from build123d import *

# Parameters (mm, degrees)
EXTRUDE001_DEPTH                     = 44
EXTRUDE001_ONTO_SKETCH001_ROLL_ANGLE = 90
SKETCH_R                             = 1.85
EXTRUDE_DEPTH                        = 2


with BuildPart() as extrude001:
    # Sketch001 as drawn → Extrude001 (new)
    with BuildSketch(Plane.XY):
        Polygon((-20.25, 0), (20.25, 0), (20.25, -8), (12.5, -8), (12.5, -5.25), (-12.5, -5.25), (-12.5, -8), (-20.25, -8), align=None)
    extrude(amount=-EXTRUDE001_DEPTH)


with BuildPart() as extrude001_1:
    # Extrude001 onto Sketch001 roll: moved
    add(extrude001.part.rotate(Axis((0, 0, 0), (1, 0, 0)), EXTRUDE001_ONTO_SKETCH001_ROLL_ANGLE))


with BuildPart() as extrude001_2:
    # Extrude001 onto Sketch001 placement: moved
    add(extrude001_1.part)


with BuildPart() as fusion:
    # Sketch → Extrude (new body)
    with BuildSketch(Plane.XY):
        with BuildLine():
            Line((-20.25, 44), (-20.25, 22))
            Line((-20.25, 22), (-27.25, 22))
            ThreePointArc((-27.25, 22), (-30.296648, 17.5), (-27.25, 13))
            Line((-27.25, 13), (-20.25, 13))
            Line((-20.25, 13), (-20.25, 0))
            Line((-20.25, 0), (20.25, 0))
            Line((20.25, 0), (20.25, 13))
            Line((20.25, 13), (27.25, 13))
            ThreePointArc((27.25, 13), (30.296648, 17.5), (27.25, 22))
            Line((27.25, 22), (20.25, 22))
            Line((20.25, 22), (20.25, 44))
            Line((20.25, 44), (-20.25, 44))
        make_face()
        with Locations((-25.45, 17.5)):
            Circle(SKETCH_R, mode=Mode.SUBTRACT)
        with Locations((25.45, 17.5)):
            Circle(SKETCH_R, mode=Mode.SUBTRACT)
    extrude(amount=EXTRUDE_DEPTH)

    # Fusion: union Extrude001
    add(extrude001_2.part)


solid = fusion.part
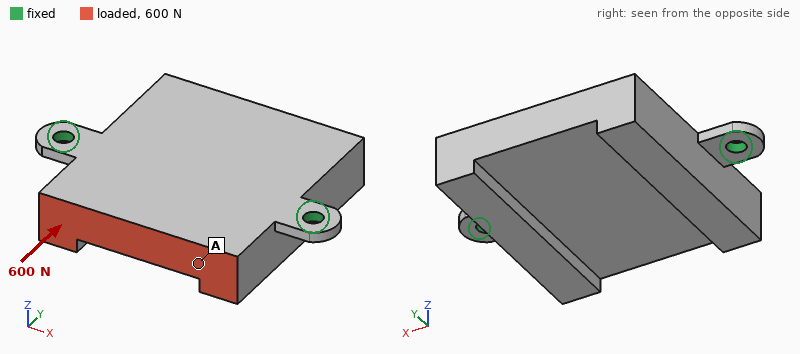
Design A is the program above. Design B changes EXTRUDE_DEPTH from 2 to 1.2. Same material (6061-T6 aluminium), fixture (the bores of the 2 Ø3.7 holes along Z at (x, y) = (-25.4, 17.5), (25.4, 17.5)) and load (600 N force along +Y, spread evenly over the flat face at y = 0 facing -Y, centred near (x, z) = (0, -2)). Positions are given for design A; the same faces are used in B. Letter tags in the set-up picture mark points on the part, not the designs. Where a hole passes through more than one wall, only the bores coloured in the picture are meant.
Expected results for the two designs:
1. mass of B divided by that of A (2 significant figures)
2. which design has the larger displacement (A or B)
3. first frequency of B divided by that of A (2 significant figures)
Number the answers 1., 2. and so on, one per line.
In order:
1. 0.90
2. B
3. 0.58
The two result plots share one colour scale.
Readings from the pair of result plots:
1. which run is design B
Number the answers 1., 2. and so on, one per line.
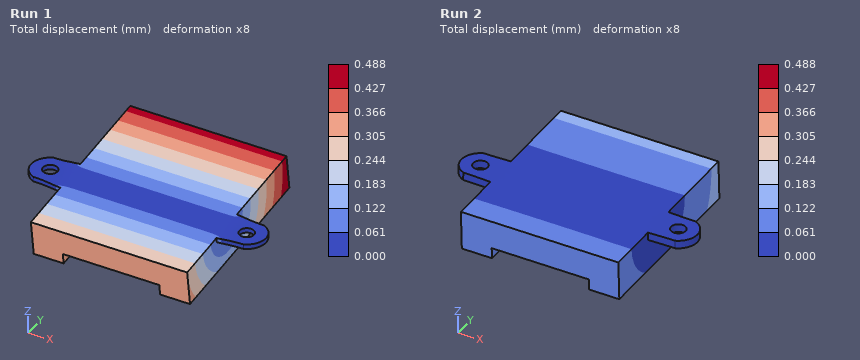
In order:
1. Run 1
